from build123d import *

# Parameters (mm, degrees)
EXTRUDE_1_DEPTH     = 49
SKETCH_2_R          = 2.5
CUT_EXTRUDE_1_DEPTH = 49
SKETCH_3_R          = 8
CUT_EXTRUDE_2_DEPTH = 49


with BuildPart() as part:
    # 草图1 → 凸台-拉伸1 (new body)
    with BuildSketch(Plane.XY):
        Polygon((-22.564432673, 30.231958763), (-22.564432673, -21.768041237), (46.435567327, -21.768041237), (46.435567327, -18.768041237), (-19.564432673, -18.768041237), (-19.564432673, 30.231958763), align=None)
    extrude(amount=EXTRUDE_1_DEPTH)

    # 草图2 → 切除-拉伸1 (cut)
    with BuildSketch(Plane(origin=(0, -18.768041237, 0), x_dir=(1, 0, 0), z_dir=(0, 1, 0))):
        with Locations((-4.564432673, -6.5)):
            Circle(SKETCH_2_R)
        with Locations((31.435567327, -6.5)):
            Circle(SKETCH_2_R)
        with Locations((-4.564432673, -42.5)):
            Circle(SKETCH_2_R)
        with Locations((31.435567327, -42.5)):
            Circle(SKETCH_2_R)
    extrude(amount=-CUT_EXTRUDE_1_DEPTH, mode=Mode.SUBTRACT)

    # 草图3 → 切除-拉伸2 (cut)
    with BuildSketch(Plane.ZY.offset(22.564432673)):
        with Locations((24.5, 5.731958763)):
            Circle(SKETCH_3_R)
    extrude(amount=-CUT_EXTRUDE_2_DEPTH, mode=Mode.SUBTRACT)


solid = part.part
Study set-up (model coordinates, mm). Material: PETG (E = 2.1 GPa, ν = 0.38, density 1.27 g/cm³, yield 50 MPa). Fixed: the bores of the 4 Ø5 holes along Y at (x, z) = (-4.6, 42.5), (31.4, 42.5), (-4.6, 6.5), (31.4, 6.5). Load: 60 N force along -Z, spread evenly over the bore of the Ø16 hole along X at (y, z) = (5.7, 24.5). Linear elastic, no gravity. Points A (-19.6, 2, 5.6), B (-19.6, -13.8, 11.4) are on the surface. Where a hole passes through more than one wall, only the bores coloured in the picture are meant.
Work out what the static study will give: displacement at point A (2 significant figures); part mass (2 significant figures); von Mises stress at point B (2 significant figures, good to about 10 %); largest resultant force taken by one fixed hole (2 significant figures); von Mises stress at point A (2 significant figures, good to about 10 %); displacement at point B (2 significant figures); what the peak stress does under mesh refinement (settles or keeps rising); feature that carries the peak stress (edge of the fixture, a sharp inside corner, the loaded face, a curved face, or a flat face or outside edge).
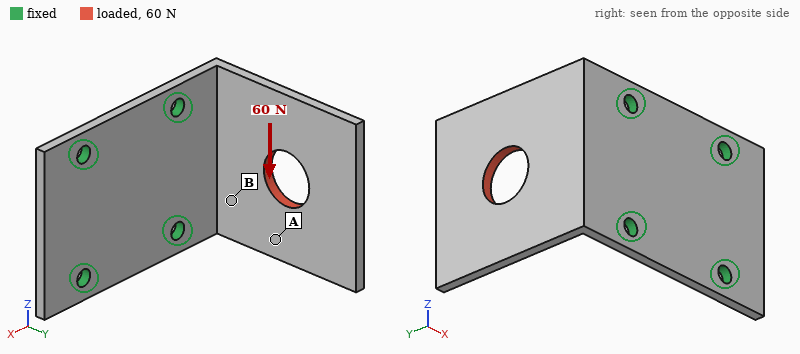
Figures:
0.57 mm
21 g
4.5 MPa
57 N
1.9 MPa
0.25 mm
keeps rising
edge of the fixture
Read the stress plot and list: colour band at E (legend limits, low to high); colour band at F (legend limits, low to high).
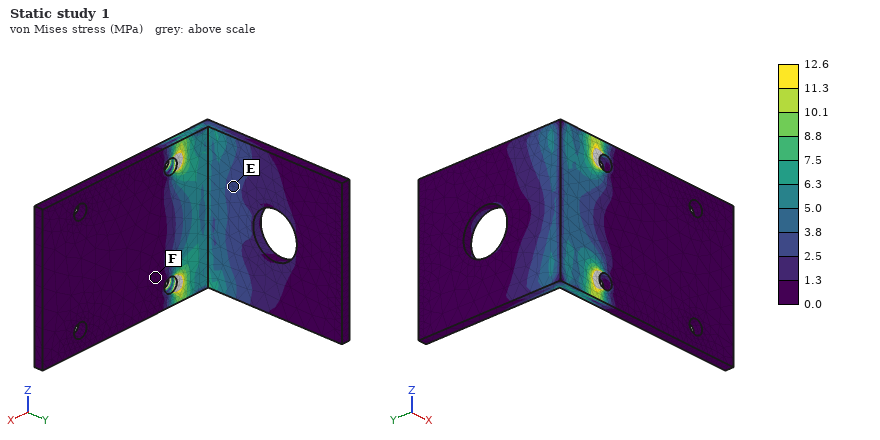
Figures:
2.5 to 3.8 MPa
0.0 to 1.3 MPa
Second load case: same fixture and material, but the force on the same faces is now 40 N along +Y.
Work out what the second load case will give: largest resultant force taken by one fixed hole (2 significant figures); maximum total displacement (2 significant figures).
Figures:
21 N
1.1 mm
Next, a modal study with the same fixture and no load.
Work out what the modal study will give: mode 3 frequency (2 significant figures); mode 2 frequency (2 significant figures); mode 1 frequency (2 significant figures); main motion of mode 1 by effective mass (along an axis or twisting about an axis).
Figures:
610 Hz
430 Hz
170 Hz
along X
